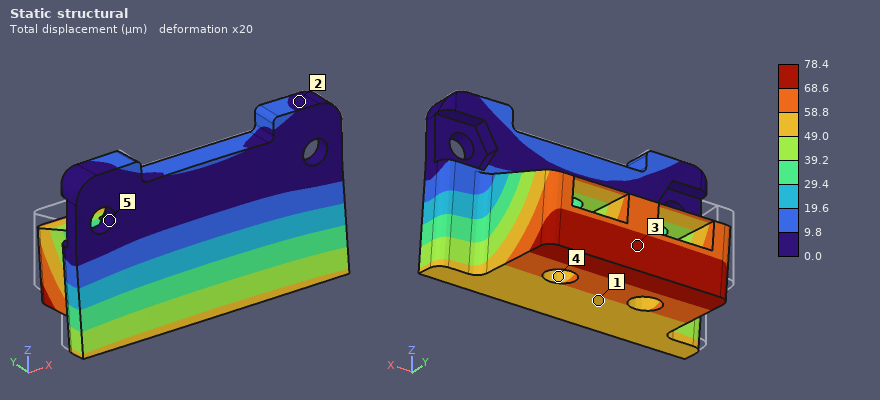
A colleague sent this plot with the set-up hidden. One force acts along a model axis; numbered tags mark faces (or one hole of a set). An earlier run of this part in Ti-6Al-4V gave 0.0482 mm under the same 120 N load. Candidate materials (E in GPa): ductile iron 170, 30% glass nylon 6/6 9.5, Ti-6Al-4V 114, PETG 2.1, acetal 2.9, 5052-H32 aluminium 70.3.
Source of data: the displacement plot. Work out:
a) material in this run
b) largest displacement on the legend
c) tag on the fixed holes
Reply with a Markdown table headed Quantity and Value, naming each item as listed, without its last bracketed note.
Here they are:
| Quantity | Value |
|---|---|
| material in this run | 5052-H32 aluminium |
| largest displacement on the legend | 78.4 µm |
| tag on the fixed holes | 5 |
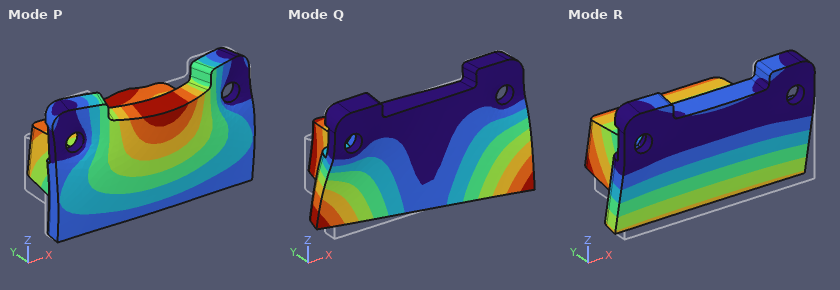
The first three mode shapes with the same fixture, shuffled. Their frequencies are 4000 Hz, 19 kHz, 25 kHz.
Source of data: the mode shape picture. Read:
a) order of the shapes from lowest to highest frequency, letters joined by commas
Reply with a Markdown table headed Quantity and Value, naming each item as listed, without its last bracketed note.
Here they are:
| Quantity | Value |
|---|---|
| order of the shapes from lowest to highest frequency, letters joined by commas | R, Q, P |
